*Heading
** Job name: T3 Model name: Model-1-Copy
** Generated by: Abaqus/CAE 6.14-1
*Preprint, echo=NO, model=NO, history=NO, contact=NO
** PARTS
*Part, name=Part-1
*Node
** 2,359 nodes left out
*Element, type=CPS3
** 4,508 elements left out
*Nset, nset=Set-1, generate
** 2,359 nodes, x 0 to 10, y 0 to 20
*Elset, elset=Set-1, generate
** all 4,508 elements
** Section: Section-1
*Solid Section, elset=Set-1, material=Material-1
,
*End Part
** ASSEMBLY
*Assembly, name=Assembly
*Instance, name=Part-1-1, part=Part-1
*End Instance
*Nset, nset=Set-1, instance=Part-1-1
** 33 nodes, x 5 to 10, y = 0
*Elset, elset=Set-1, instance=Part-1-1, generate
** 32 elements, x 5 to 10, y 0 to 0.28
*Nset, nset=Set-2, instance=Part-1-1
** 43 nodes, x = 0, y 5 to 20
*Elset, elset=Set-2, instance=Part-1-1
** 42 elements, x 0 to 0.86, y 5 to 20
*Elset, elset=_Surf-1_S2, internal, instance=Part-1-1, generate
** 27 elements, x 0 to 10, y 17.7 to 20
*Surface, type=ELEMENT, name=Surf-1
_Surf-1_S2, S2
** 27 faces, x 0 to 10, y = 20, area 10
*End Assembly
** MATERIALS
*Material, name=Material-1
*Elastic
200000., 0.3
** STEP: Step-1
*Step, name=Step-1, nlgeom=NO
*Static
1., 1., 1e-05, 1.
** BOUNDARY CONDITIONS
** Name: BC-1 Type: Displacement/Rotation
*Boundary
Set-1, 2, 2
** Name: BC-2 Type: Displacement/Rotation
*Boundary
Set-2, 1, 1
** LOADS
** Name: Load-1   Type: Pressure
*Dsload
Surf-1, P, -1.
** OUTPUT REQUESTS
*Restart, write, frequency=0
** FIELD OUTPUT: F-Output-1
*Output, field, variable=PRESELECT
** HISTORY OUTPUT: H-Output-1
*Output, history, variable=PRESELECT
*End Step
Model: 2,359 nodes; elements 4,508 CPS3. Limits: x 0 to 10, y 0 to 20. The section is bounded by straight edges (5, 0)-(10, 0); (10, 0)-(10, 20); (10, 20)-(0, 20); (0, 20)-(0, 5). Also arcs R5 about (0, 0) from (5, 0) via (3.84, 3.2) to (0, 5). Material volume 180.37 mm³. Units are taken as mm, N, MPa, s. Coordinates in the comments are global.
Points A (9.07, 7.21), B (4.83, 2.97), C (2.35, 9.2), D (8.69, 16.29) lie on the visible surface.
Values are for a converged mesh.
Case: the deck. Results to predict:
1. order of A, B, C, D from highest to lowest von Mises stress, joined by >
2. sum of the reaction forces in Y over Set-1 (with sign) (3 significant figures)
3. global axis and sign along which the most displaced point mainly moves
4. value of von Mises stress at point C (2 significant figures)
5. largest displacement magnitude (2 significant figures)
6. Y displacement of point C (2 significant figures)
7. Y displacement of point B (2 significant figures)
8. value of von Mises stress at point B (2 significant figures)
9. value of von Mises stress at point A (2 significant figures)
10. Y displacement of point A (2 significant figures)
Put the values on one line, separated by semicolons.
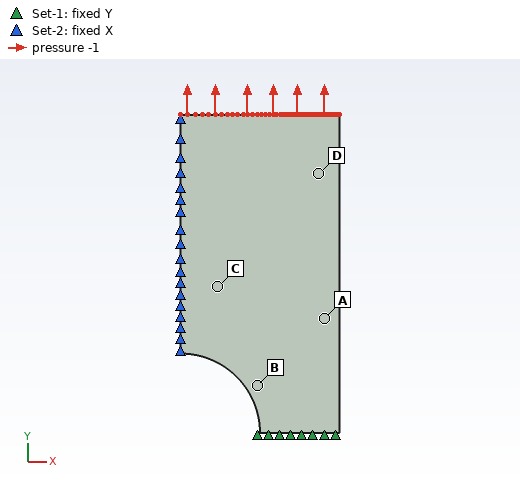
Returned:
B > A > D > C; -10.0 N; +Y; 0.72 MPa; 1.5e-04 mm; 1.0e-04 mm; 4.8e-05 mm; 1.9 MPa; 1.7 MPa; 5.3e-05 mm
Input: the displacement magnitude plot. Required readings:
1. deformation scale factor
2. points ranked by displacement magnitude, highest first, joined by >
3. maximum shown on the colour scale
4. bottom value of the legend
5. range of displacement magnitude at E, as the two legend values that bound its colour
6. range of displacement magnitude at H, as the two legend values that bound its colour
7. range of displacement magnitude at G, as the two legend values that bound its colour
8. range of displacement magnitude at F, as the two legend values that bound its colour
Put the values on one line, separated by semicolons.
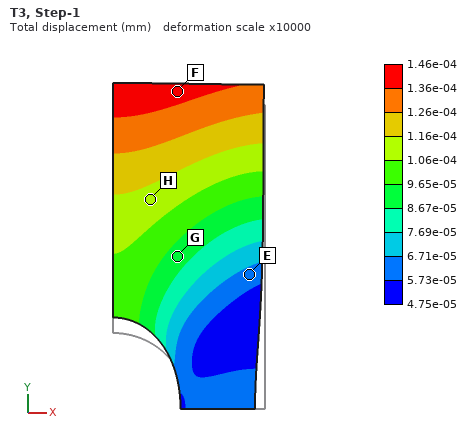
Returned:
10000; F > H > G > E; 1.46e-04 mm; 4.75e-05 mm; 5.73e-05 to 6.71e-05 mm; 1.06e-04 to 1.16e-04 mm; 8.67e-05 to 9.65e-05 mm; 1.36e-04 to 1.46e-04 mm
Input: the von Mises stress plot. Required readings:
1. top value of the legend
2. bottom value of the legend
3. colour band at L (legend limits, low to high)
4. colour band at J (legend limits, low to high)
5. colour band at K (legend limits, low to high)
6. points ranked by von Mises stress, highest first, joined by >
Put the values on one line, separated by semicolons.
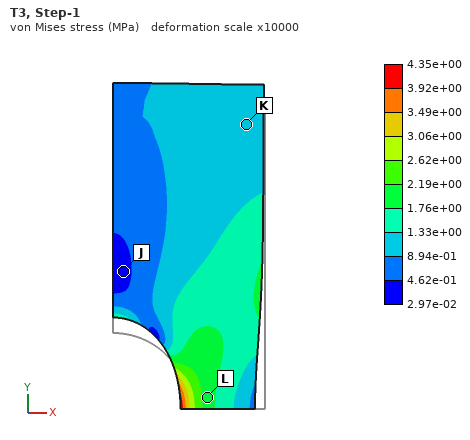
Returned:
4.35e+00 MPa; 2.97e-02 MPa; 1.76e+00 to 2.19e+00 MPa; 2.97e-02 to 4.62e-01 MPa; 8.94e-01 to 1.33e+00 MPa; L > K > J
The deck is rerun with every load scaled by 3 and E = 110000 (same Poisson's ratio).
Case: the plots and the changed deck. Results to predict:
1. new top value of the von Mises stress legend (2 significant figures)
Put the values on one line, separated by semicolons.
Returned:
13 MPa
